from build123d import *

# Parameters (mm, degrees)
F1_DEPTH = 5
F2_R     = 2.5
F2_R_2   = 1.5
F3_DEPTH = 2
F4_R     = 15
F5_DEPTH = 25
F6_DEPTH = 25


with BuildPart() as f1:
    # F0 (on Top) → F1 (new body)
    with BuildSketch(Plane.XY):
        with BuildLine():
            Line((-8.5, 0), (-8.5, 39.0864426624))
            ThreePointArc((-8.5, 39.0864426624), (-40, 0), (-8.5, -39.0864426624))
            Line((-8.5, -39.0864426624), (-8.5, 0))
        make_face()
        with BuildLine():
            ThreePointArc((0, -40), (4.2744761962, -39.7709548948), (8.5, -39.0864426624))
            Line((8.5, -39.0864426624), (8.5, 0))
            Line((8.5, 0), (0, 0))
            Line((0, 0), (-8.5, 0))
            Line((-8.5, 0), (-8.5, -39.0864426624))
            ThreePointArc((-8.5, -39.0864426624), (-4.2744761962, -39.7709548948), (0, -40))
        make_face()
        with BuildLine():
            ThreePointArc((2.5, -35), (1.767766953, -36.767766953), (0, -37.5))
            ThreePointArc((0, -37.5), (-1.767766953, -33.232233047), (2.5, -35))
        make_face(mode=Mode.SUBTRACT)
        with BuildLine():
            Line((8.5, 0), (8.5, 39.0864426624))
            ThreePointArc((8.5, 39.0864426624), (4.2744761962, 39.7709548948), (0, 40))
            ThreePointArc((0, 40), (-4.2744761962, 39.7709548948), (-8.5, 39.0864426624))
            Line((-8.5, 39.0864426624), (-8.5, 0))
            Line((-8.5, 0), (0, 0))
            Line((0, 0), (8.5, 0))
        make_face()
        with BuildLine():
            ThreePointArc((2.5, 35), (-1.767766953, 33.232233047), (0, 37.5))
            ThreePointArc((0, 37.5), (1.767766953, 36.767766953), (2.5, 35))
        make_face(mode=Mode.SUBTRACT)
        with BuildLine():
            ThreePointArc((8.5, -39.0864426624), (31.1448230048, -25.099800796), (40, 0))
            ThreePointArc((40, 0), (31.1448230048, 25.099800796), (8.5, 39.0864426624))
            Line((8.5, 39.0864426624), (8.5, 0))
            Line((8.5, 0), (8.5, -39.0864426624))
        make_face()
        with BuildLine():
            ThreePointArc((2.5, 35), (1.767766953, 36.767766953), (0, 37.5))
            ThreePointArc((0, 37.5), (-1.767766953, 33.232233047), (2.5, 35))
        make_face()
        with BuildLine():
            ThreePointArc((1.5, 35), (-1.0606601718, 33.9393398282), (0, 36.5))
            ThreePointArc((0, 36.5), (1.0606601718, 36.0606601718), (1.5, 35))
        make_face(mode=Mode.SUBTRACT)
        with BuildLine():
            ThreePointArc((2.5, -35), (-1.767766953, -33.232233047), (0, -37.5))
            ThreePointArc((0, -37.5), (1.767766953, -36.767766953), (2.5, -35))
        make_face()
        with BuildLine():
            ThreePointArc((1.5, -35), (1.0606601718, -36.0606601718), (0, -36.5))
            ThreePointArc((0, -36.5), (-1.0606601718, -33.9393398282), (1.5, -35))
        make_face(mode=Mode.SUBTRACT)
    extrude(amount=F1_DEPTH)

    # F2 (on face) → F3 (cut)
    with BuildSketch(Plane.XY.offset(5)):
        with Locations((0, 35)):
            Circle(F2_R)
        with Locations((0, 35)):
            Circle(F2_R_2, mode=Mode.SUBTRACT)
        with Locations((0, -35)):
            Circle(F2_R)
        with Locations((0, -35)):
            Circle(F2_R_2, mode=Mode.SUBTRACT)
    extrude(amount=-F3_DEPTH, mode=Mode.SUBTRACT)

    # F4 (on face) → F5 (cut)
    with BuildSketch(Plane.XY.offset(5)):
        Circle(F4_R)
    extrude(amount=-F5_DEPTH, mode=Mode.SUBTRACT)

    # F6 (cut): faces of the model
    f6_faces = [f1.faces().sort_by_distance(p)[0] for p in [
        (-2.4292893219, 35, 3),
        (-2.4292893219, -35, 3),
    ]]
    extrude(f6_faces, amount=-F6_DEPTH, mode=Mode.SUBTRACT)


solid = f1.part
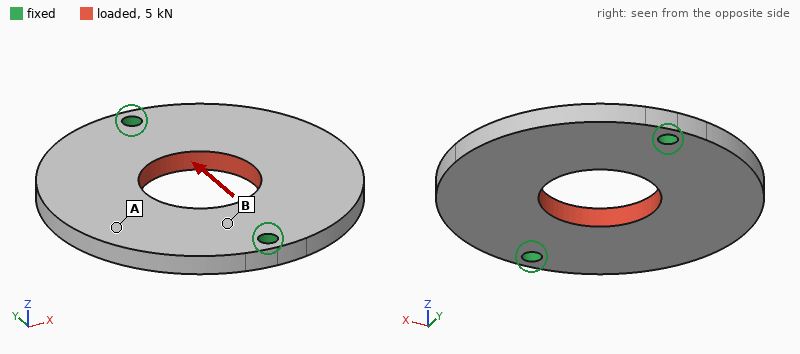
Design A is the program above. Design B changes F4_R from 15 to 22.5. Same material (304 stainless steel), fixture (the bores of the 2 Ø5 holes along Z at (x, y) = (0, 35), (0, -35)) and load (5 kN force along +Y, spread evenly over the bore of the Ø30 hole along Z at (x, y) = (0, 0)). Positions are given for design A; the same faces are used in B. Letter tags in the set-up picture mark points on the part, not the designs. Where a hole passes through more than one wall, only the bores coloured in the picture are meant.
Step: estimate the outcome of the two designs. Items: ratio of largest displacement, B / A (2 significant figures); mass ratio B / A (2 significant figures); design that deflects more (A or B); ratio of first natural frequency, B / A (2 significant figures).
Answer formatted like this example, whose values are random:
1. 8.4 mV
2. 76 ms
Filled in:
1. 1.7
2. 0.79
3. B
4. 0.99
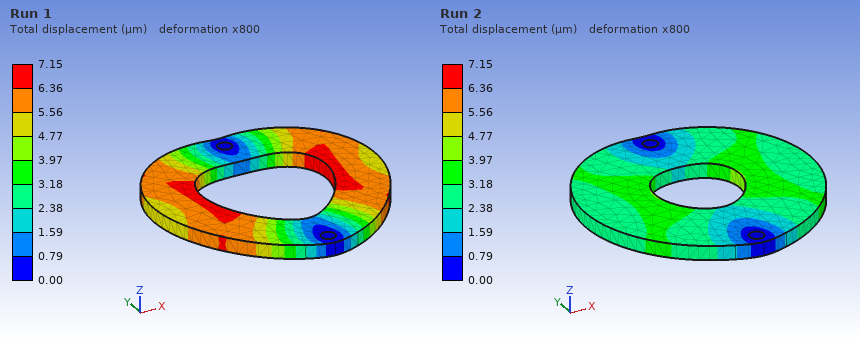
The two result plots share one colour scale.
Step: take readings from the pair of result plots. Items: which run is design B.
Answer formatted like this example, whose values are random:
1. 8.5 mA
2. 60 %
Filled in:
1. Run 1
